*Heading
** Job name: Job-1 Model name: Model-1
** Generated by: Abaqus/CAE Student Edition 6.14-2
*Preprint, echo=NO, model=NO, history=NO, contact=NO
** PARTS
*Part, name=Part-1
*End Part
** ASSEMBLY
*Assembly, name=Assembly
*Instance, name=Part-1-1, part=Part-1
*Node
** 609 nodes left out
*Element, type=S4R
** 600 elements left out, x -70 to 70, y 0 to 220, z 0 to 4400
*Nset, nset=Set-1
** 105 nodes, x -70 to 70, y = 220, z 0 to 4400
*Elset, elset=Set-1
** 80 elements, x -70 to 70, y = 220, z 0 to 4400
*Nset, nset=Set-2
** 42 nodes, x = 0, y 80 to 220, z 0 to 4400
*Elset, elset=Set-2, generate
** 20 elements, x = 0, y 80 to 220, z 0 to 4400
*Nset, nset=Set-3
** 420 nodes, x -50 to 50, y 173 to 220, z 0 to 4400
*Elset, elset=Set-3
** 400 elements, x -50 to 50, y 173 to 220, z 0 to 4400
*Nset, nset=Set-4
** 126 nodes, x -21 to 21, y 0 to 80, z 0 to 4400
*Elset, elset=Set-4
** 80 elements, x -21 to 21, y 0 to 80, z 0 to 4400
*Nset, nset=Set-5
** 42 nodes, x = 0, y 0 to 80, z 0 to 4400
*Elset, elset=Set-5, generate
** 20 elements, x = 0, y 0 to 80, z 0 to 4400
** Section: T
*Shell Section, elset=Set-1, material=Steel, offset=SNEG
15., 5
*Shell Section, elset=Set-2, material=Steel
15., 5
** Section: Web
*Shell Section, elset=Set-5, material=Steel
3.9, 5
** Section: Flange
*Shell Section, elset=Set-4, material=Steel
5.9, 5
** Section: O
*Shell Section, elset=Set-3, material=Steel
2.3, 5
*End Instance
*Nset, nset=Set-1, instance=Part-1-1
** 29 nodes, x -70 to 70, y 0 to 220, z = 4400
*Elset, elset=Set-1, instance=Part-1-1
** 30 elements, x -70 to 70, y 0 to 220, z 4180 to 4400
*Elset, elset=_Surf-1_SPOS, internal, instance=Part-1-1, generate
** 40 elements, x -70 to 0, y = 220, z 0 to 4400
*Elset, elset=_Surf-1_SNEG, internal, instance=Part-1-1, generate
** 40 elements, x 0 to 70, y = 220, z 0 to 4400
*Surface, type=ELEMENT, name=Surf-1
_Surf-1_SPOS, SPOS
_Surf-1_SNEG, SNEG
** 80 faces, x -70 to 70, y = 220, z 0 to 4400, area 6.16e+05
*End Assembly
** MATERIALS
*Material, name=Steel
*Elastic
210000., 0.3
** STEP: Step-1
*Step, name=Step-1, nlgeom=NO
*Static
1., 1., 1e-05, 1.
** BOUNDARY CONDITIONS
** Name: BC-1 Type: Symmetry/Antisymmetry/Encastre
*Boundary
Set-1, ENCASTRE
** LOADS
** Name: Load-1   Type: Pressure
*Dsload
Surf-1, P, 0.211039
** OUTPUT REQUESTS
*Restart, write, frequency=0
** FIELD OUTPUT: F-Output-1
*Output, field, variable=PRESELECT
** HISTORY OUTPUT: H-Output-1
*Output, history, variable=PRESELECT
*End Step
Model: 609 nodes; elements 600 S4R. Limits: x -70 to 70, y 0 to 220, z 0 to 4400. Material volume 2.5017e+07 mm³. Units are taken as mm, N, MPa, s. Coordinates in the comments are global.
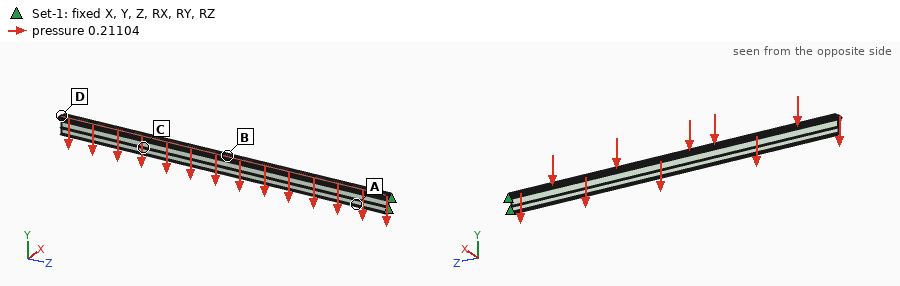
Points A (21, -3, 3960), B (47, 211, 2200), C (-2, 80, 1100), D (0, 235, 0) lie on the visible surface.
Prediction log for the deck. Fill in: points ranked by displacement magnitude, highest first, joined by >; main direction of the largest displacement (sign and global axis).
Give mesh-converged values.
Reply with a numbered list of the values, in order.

1. D > C > B > A
2. -Y
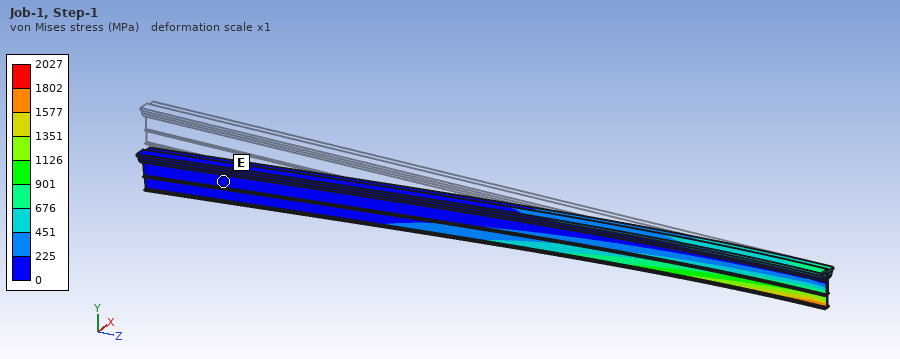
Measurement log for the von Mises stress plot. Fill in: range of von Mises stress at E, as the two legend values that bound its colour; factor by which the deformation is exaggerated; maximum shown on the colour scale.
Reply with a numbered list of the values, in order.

1. 0 to 225 MPa
2. 1
3. 2027 MPa
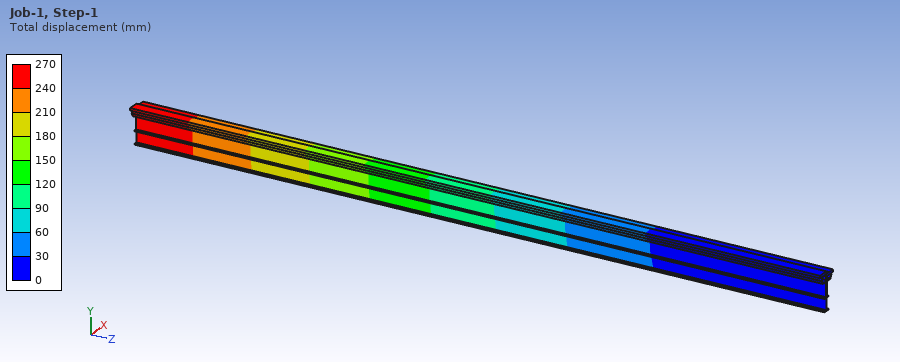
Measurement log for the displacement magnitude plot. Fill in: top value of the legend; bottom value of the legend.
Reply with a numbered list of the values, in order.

1. 270 mm
2. 0 mm
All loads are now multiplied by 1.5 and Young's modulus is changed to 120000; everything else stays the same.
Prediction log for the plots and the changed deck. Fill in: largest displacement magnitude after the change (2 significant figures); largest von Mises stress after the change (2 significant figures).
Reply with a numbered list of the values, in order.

1. 710 mm
2. 3000 MPa
